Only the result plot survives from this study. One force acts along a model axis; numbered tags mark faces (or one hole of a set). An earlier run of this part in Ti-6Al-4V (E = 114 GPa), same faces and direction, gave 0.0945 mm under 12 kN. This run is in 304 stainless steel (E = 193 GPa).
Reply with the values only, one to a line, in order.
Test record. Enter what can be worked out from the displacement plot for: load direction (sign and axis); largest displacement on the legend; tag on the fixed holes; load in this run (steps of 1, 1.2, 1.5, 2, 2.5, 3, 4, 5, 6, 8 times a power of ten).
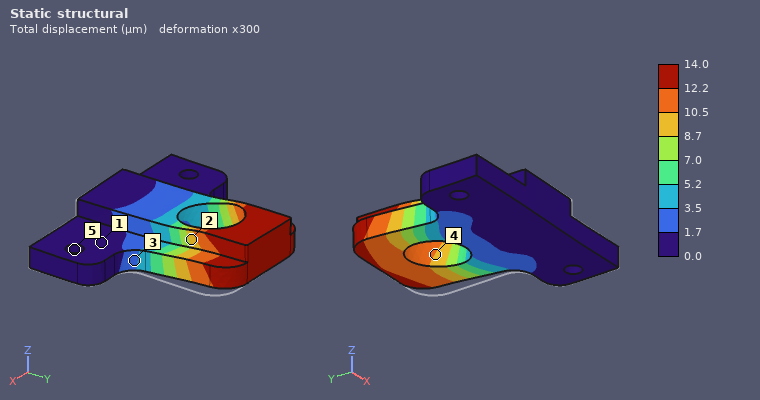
-X
14.0 µm
5
3 kN
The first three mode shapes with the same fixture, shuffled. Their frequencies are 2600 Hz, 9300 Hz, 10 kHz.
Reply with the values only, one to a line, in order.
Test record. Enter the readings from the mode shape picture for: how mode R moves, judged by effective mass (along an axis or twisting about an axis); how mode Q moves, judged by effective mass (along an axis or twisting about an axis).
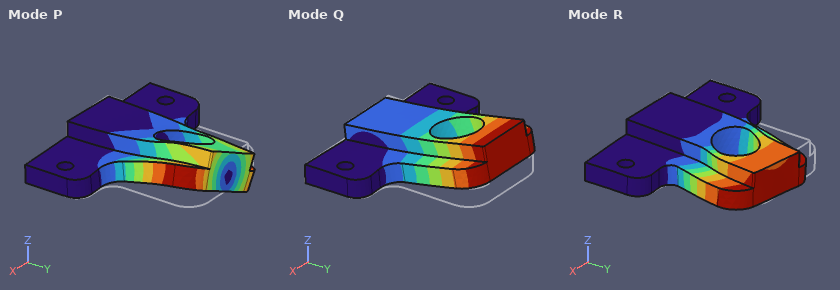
along X
along Z
